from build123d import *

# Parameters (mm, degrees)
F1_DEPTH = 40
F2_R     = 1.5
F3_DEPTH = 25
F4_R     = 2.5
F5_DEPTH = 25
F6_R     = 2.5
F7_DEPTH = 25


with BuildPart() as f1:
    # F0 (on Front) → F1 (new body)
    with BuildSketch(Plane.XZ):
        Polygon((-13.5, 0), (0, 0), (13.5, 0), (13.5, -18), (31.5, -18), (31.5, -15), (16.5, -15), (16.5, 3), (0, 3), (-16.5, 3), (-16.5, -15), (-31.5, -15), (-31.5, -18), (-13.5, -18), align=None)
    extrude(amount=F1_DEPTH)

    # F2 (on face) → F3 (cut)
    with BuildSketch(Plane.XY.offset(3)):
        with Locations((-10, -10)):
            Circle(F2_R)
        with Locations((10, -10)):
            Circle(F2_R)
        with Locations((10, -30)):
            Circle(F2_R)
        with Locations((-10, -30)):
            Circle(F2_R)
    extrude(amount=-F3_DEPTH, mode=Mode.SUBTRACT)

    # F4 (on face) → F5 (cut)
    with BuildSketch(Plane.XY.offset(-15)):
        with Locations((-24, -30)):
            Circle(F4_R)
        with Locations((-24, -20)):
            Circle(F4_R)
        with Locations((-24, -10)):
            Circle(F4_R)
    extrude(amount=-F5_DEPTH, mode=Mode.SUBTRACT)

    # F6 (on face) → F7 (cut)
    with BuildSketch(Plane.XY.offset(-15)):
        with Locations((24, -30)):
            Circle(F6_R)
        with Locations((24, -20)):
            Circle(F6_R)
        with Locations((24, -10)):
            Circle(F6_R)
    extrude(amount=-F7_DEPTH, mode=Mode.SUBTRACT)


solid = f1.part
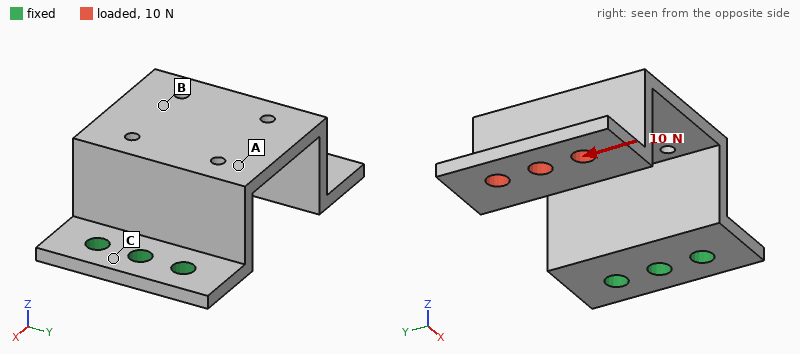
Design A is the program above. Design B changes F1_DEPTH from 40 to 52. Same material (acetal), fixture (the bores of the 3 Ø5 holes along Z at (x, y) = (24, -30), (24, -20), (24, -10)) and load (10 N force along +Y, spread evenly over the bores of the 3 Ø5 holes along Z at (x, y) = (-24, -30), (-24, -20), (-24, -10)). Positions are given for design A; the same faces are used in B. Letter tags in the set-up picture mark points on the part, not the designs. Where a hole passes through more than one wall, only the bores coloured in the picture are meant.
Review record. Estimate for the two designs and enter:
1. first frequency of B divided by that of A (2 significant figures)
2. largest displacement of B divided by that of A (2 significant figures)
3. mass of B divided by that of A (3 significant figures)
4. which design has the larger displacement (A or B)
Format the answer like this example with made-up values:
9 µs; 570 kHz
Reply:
0.97; 0.75; 1.31; A
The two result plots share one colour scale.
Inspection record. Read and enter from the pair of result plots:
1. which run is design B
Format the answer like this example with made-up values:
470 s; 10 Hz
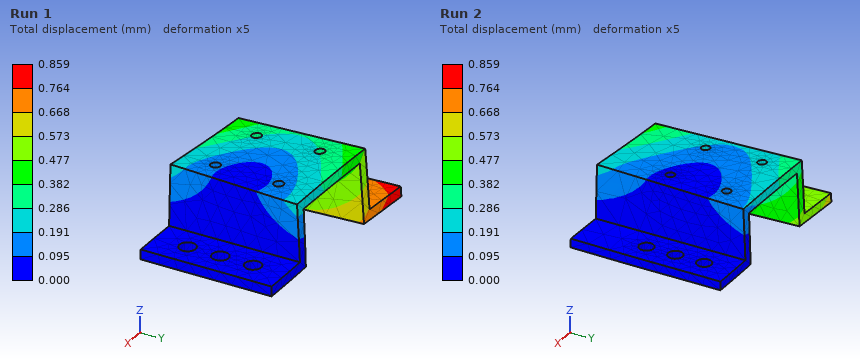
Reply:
Run 2
